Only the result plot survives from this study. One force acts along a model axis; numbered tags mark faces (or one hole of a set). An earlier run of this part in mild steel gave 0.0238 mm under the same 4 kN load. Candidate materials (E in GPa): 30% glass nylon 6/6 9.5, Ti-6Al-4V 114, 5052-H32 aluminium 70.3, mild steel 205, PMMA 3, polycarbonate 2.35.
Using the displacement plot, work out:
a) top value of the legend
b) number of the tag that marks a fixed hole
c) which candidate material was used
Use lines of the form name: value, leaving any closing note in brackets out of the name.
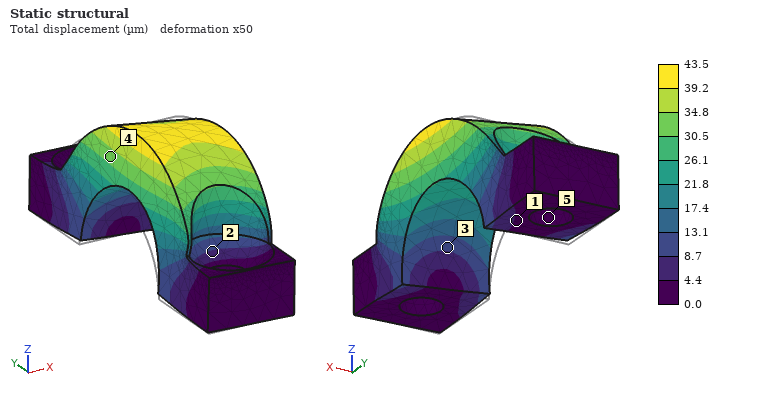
top value of the legend: 43.5 µm
number of the tag that marks a fixed hole: 5
which candidate material was used: Ti-6Al-4V
